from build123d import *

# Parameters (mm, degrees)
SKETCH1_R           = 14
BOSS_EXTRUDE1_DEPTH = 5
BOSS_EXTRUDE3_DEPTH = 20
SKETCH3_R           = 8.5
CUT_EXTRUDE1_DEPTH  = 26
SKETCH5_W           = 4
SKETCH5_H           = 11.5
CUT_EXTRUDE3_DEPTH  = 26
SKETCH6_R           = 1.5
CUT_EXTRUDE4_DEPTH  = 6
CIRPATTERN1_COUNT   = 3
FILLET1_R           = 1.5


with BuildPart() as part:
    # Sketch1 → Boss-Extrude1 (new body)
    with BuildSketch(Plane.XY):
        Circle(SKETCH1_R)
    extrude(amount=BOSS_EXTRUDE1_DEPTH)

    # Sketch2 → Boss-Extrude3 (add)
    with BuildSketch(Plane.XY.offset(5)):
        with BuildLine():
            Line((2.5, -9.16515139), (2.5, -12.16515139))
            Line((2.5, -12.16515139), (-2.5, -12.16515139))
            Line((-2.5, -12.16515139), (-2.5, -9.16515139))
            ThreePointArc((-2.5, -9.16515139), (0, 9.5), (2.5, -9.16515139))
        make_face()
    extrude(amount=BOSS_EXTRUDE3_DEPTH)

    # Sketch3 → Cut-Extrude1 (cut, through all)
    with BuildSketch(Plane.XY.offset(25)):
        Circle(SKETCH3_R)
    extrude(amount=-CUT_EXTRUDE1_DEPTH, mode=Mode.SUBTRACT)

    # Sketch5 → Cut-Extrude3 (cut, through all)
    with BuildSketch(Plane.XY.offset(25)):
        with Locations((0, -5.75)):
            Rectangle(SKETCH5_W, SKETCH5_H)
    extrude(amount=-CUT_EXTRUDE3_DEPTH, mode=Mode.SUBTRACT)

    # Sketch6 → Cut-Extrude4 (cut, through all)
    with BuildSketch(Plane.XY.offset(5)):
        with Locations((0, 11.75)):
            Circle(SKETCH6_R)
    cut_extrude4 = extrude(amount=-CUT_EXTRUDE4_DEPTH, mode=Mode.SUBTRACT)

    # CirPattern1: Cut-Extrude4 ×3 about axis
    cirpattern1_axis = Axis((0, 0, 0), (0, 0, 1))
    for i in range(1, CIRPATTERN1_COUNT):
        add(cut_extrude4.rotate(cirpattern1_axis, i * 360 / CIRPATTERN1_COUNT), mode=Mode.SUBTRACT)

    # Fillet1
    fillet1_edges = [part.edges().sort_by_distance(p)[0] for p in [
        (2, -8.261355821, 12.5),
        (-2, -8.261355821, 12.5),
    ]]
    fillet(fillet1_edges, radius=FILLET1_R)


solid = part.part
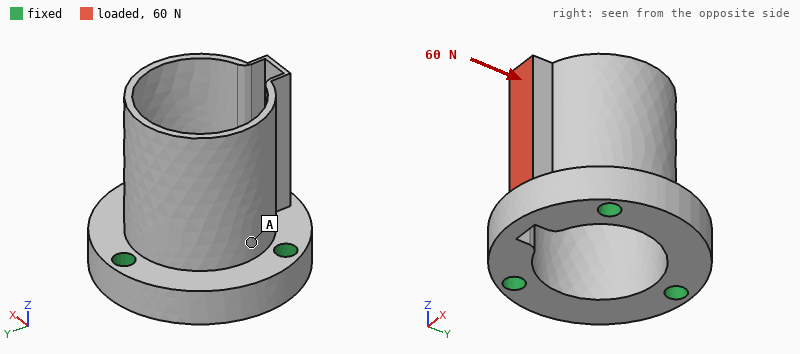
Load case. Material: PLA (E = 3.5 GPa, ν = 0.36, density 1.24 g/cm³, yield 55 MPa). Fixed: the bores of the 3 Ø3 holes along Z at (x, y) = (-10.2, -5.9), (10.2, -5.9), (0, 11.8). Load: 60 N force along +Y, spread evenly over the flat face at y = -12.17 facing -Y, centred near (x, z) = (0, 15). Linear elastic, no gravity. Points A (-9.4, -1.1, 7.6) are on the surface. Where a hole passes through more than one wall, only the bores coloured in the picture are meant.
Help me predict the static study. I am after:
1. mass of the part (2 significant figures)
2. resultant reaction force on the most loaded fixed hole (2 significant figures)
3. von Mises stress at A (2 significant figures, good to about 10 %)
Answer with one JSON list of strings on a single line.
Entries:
["3.6 g", "36 N", "3.7 MPa"]
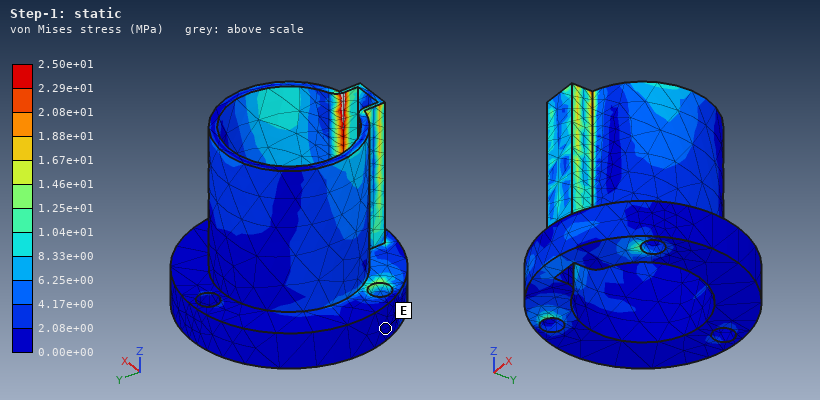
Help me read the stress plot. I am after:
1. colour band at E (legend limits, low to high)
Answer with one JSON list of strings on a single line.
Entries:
["0.00e+00 to 2.08e+00 MPa"]
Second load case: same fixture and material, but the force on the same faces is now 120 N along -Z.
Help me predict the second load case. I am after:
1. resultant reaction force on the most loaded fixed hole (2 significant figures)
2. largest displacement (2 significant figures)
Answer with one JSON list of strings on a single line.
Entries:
["68 N", "0.25 mm"]
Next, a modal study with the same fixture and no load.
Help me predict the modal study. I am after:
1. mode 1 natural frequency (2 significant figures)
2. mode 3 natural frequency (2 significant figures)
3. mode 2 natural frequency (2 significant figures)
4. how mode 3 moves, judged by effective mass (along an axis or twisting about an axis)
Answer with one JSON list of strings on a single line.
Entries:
["3100 Hz", "4800 Hz", "4100 Hz", "along Y"]
